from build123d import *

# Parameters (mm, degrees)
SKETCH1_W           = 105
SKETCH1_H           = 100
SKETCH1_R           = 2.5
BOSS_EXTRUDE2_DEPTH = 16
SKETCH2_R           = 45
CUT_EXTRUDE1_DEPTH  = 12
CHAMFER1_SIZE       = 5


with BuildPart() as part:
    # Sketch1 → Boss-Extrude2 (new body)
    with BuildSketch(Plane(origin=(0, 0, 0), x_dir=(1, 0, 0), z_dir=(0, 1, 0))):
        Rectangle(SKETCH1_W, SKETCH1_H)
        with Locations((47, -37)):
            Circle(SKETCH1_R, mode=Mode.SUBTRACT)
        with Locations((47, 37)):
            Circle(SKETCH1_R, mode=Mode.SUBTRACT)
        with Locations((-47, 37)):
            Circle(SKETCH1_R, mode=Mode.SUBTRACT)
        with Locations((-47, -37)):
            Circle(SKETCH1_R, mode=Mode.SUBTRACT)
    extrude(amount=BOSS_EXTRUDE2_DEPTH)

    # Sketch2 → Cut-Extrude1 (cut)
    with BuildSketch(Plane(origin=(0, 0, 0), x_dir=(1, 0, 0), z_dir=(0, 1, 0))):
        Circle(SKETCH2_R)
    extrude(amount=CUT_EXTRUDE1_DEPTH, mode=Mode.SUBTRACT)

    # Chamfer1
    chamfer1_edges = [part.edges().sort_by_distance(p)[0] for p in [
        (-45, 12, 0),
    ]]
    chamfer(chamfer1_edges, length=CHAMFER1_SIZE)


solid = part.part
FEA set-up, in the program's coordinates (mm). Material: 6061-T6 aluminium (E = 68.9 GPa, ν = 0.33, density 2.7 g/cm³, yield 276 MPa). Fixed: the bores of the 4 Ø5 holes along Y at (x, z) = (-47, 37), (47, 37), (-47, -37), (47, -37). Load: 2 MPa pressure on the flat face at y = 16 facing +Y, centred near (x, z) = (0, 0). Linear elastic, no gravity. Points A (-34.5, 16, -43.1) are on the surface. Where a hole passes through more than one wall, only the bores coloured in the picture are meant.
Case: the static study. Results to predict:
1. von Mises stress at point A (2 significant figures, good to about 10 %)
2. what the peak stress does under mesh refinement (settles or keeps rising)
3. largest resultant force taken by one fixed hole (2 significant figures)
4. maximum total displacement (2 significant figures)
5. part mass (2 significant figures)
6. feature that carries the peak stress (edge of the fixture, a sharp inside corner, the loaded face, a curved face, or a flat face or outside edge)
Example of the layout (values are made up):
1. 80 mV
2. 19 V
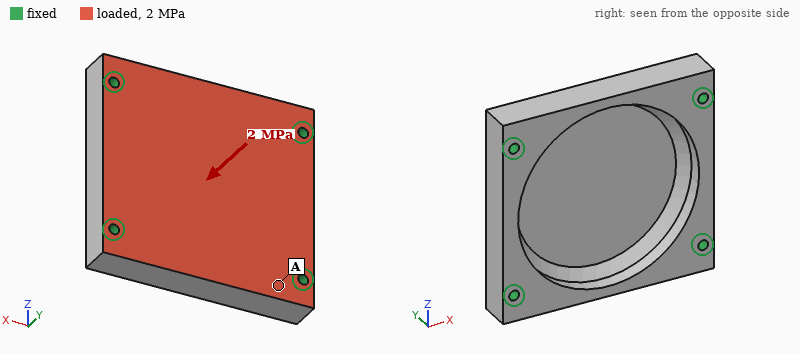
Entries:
1. 20 MPa
2. keeps rising
3. 6.0 kN
4. 0.33 mm
5. 250 g
6. edge of the fixture
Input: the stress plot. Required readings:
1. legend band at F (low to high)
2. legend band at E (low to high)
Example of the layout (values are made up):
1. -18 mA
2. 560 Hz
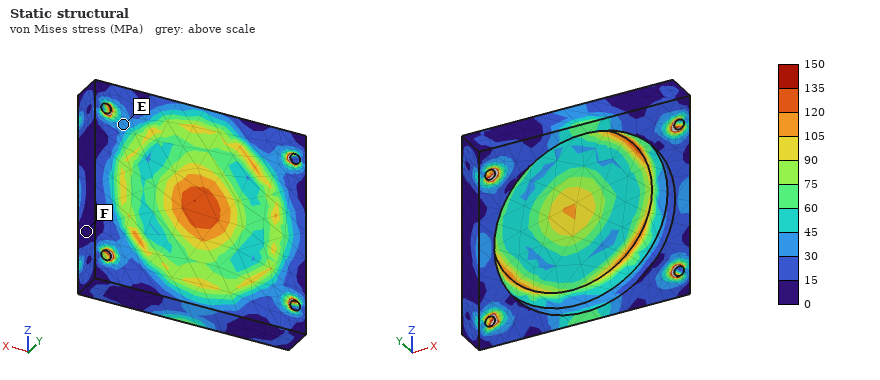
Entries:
1. 0 to 15 MPa
2. 30 to 45 MPa
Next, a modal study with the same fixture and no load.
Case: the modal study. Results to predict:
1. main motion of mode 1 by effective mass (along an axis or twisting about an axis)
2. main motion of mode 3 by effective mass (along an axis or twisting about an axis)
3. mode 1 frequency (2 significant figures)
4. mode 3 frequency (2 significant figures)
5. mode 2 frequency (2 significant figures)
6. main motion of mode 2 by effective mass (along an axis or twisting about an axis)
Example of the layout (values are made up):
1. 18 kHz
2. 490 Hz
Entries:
1. along Y
2. along Y
3. 4800 Hz
4. 8900 Hz
5. 7800 Hz
6. twisting about X
